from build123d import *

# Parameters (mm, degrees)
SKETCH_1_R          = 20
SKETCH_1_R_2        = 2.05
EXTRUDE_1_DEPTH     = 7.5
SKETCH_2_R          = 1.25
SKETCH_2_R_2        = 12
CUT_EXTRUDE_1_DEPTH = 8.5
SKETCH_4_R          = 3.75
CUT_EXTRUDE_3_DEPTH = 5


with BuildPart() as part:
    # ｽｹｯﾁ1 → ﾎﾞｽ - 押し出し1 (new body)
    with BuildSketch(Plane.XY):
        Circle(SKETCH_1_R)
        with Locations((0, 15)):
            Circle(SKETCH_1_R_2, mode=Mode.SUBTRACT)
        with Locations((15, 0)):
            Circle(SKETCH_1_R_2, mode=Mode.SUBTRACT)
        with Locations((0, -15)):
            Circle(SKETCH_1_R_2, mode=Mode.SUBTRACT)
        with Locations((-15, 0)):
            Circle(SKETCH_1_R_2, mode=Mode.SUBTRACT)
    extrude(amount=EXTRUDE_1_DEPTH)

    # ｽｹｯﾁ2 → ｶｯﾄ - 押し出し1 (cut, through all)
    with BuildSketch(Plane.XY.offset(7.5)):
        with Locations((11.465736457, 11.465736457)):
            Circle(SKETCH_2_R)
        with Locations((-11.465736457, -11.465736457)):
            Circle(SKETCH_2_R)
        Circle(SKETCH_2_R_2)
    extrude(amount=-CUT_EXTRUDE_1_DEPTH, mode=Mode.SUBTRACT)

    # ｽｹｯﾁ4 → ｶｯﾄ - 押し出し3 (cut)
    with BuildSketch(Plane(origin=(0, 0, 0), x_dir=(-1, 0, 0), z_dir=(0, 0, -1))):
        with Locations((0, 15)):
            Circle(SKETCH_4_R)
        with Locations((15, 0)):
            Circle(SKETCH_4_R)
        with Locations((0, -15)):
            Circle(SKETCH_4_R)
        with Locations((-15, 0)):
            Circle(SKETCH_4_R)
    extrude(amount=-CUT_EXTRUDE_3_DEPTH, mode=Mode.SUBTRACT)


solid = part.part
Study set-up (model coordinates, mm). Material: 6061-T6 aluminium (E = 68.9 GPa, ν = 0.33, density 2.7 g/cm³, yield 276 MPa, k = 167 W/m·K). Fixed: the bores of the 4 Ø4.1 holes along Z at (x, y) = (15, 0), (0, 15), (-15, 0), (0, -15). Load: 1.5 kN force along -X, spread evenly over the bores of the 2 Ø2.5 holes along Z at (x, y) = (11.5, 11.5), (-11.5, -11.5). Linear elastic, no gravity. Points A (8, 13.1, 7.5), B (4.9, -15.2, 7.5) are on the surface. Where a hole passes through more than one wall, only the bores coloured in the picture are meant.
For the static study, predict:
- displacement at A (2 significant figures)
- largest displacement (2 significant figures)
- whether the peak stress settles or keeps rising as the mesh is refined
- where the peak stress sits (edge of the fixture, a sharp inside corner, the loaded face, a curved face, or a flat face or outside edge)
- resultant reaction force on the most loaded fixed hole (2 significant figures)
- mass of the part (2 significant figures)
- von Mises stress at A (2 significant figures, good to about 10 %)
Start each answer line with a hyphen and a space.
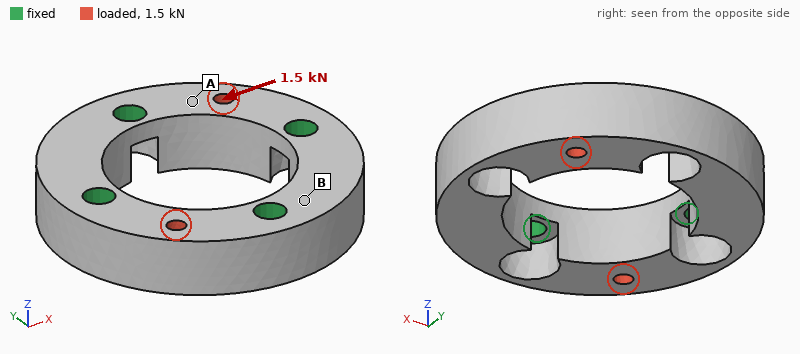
- 3.2 µm
- 13 µm
- keeps rising
- a sharp inside corner
- 580 N
- 13 g
- 20 MPa
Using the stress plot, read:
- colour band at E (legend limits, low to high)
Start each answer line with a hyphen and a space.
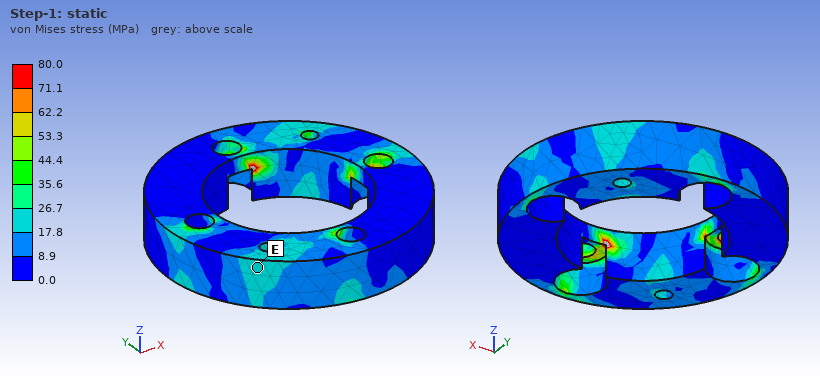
- 17.8 to 26.7 MPa
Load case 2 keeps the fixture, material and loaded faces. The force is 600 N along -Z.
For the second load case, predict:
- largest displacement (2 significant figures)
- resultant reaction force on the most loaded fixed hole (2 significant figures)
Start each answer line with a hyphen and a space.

- 13 µm
- 160 N
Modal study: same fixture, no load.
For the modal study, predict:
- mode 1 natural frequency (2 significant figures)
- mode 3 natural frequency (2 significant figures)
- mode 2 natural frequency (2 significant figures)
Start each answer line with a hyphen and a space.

- 16 kHz
- 19 kHz
- 19 kHz
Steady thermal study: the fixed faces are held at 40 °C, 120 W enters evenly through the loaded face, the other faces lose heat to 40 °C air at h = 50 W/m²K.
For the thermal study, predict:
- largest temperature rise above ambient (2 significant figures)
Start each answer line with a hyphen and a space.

- 53 K
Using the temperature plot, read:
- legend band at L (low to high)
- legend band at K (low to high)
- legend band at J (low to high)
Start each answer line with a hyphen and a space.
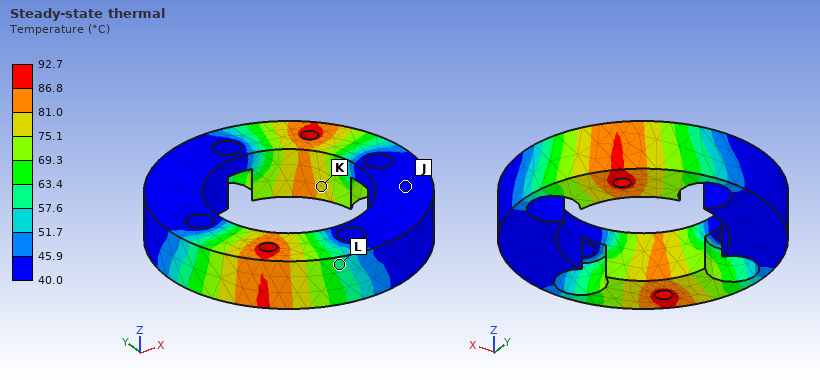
- 57.6 to 63.4 °C
- 75.1 to 81.0 °C
- 40.0 to 45.9 °C
